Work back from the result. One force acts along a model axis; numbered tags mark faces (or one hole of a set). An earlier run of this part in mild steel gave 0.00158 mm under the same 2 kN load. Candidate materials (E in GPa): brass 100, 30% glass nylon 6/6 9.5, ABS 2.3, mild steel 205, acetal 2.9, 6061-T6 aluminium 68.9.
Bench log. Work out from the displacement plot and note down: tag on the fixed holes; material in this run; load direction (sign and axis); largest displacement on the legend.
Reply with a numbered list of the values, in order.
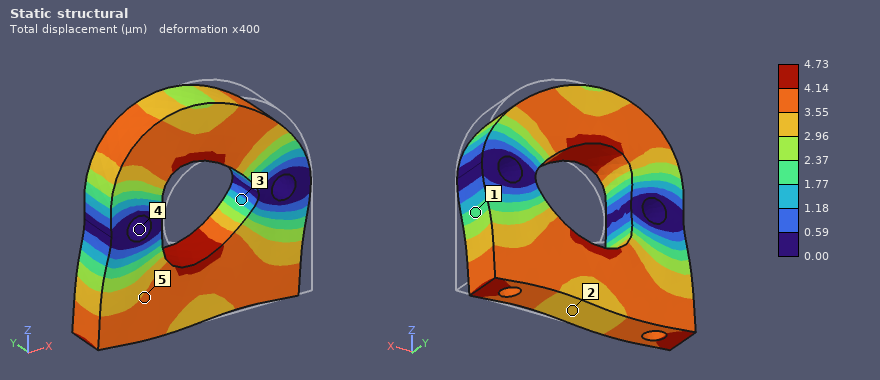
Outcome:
1. 4
2. 6061-T6 aluminium
3. -X
4. 4.73 µm
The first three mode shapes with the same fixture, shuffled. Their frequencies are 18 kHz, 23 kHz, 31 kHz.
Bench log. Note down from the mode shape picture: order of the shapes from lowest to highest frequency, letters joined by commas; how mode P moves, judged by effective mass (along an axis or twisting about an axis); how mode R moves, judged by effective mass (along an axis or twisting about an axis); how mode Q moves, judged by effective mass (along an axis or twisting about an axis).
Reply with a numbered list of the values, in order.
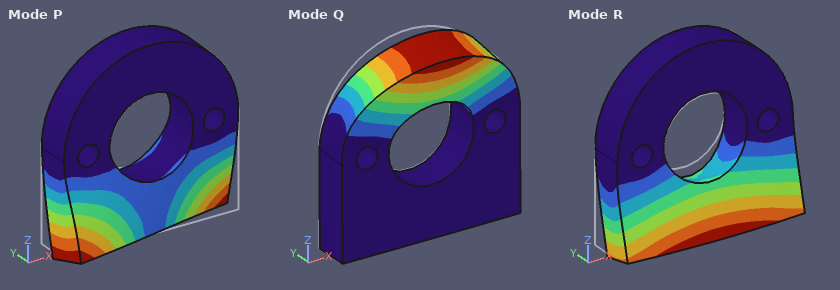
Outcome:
1. R, Q, P
2. twisting about Z
3. along Y
4. along Y
